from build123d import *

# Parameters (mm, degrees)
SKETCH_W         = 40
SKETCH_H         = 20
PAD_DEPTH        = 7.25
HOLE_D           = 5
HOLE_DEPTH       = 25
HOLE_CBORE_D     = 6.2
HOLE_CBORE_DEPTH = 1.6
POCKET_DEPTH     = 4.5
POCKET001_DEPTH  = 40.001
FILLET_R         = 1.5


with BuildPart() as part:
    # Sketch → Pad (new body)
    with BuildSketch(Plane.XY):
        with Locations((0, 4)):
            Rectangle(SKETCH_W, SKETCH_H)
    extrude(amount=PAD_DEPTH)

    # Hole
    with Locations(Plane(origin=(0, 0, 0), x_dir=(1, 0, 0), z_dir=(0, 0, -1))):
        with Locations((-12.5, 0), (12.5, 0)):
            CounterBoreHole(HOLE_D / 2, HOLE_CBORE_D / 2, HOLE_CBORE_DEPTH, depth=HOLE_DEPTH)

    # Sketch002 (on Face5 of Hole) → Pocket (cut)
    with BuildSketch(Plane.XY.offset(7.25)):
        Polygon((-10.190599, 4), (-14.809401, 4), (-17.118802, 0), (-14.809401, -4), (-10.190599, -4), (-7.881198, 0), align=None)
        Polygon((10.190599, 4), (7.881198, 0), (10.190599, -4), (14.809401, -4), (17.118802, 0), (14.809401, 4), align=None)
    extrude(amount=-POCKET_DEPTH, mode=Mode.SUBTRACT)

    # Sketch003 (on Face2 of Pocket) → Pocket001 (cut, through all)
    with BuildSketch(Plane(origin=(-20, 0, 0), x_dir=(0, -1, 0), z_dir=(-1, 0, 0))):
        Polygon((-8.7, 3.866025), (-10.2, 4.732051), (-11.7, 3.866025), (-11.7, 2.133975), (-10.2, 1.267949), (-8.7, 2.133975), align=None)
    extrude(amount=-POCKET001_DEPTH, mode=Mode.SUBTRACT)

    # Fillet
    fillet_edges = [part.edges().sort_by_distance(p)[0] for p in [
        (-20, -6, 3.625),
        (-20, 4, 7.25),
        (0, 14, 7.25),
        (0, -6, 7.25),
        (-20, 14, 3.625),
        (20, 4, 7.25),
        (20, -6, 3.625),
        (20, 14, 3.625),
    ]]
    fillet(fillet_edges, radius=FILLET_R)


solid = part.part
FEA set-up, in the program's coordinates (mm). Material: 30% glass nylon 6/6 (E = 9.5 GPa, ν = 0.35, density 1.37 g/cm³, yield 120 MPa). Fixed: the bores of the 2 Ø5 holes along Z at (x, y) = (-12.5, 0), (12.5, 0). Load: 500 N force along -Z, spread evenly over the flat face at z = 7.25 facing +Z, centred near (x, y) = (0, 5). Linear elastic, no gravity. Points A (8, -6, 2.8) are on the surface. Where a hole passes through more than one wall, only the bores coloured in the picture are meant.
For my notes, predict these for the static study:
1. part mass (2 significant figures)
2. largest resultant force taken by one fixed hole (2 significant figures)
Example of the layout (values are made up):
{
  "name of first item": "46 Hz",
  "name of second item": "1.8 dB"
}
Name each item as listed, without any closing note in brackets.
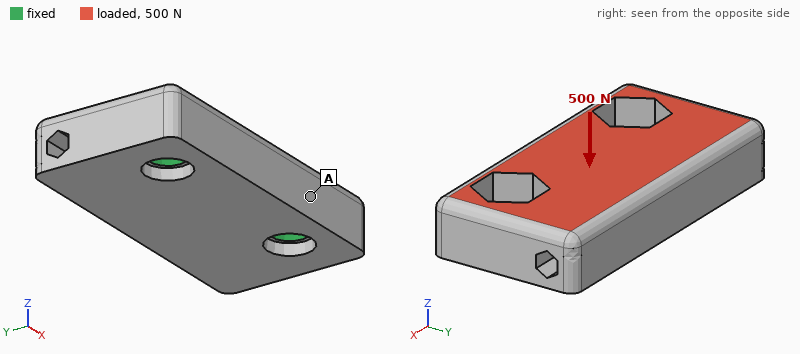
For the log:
{
  "part mass": "6.5 g",
  "largest resultant force taken by one fixed hole": "250 N"
}
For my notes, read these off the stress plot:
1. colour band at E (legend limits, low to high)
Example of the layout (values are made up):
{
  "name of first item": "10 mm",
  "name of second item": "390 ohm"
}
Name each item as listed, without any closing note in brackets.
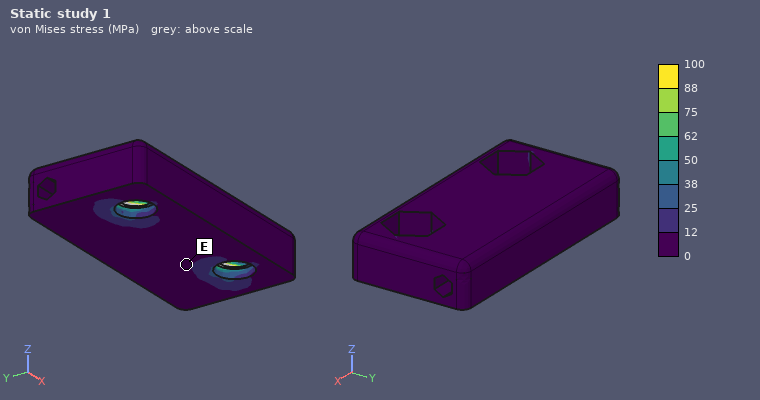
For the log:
{
  "colour band at E": "0 to 12 MPa"
}
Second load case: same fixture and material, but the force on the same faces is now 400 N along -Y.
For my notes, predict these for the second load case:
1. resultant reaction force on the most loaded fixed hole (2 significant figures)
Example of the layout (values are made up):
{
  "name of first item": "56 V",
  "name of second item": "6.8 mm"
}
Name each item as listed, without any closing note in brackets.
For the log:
{
  "resultant reaction force on the most loaded fixed hole": "200 N"
}
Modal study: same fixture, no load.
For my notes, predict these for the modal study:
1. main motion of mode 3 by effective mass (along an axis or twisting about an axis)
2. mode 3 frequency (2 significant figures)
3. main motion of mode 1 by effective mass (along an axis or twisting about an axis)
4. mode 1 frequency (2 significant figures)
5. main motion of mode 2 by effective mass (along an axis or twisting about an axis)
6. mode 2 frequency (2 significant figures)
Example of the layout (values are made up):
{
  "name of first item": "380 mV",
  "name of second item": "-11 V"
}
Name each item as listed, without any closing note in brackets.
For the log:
{
  "main motion of mode 3 by effective mass": "along Z",
  "mode 3 frequency": "12 kHz",
  "main motion of mode 1 by effective mass": "along Z",
  "mode 1 frequency": "4200 Hz",
  "main motion of mode 2 by effective mass": "twisting about Y",
  "mode 2 frequency": "9600 Hz"
}
